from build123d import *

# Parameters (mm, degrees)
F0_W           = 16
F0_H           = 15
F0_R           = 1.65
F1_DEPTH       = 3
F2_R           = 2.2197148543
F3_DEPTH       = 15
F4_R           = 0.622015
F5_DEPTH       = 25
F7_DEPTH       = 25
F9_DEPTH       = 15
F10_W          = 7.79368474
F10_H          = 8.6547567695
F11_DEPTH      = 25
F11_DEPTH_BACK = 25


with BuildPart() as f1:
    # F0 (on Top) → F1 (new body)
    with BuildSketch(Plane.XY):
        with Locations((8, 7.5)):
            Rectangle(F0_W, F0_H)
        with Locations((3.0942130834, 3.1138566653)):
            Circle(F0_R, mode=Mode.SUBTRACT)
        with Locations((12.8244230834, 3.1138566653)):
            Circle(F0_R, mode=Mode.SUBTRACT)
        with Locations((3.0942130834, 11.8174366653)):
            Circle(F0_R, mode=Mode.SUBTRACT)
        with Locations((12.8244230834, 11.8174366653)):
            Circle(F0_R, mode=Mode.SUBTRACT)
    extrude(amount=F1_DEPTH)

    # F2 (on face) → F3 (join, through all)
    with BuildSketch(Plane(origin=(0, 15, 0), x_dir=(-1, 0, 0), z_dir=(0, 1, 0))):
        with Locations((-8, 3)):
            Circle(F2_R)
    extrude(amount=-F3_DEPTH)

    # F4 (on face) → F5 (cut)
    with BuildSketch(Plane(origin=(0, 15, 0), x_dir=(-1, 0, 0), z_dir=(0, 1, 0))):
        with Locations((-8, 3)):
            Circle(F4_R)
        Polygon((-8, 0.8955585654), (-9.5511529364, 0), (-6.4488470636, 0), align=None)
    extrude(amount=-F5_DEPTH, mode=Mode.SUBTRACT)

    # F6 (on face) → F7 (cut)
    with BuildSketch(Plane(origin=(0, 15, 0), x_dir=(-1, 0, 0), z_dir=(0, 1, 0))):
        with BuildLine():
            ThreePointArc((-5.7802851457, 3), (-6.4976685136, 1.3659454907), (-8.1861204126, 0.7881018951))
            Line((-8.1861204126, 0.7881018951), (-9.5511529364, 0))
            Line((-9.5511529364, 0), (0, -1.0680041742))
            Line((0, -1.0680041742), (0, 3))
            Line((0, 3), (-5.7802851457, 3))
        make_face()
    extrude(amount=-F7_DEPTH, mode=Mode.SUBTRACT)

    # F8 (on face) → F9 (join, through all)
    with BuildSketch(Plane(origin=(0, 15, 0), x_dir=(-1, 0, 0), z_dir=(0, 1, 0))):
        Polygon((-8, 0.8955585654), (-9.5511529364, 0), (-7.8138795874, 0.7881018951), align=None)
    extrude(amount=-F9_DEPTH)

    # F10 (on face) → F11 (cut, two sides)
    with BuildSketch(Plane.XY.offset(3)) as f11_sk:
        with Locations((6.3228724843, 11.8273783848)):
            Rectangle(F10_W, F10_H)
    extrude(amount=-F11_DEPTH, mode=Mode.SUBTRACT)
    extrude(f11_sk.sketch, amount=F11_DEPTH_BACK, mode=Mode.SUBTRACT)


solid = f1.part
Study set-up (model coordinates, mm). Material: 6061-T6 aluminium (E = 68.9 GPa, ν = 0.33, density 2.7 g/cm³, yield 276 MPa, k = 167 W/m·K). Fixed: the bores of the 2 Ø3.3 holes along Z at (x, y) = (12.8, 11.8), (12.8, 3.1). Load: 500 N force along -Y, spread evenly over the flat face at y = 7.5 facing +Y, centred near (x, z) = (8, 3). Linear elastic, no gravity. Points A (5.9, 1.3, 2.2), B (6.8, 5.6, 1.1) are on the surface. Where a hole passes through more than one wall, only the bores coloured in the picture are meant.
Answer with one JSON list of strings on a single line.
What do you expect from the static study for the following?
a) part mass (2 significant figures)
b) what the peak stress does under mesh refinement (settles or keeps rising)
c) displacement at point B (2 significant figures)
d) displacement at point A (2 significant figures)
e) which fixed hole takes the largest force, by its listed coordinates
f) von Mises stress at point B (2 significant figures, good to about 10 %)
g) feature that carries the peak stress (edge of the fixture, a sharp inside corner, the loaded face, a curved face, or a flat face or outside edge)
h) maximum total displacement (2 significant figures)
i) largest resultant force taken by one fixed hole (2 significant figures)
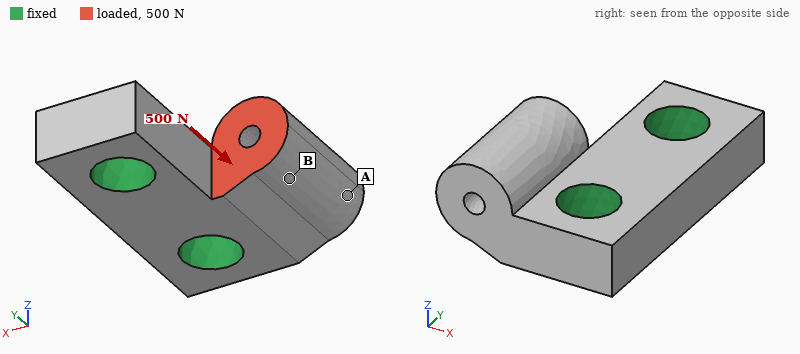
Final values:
["0.90 g", "keeps rising", "5.8 µm", "6.4 µm", "(12.8, 3.1)", "29 MPa", "a sharp inside corner", "9.9 µm", "390 N"]
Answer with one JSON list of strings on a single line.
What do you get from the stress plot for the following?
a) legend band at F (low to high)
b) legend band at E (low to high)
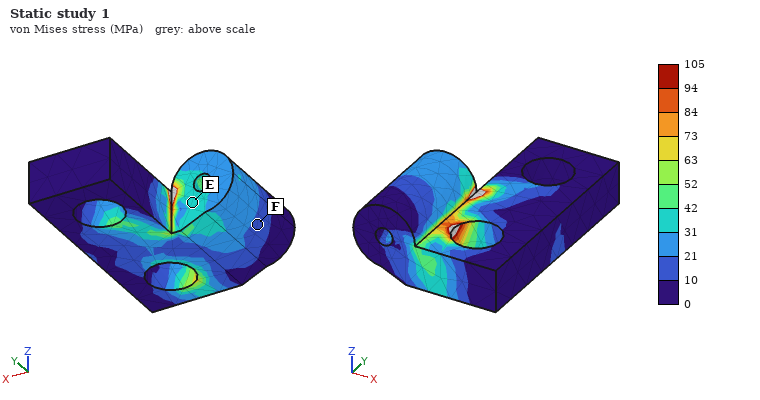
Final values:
["10 to 21 MPa", "31 to 42 MPa"]
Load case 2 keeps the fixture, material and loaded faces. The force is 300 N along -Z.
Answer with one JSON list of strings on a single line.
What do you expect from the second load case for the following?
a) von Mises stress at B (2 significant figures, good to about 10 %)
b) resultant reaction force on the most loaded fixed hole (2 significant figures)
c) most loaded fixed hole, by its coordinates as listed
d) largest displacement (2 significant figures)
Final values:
["38 MPa", "210 N", "(12.8, 3.1)", "21 µm"]
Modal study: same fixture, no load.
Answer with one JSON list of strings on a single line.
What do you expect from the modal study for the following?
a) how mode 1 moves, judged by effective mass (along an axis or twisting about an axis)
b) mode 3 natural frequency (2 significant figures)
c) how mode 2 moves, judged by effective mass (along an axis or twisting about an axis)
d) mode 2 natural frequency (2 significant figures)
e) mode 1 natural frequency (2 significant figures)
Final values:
["along Z", "91 kHz", "along Y", "75 kHz", "50 kHz"]
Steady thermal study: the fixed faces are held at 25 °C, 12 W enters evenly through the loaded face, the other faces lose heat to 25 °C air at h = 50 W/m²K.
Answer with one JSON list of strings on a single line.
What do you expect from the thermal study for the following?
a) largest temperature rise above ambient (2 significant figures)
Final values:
["22 K"]
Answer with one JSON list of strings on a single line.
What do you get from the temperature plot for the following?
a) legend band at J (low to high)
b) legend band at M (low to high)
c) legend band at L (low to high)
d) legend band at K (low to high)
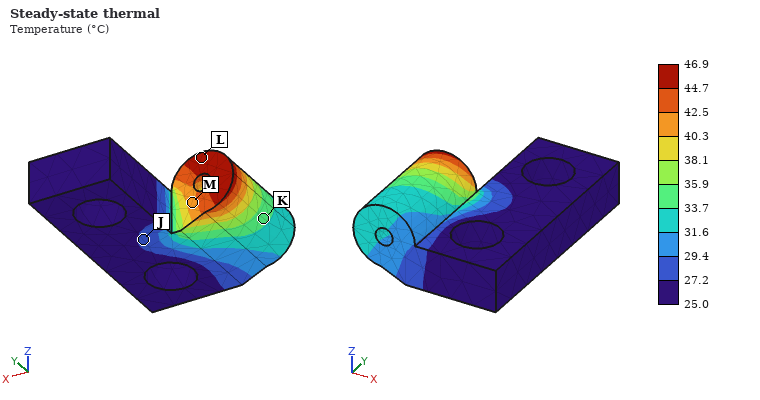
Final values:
["27.2 to 29.4 °C", "40.3 to 42.5 °C", "44.7 to 46.9 °C", "33.7 to 35.9 °C"]
